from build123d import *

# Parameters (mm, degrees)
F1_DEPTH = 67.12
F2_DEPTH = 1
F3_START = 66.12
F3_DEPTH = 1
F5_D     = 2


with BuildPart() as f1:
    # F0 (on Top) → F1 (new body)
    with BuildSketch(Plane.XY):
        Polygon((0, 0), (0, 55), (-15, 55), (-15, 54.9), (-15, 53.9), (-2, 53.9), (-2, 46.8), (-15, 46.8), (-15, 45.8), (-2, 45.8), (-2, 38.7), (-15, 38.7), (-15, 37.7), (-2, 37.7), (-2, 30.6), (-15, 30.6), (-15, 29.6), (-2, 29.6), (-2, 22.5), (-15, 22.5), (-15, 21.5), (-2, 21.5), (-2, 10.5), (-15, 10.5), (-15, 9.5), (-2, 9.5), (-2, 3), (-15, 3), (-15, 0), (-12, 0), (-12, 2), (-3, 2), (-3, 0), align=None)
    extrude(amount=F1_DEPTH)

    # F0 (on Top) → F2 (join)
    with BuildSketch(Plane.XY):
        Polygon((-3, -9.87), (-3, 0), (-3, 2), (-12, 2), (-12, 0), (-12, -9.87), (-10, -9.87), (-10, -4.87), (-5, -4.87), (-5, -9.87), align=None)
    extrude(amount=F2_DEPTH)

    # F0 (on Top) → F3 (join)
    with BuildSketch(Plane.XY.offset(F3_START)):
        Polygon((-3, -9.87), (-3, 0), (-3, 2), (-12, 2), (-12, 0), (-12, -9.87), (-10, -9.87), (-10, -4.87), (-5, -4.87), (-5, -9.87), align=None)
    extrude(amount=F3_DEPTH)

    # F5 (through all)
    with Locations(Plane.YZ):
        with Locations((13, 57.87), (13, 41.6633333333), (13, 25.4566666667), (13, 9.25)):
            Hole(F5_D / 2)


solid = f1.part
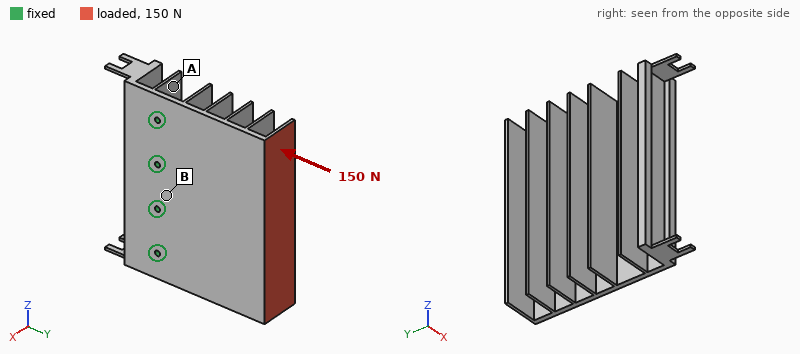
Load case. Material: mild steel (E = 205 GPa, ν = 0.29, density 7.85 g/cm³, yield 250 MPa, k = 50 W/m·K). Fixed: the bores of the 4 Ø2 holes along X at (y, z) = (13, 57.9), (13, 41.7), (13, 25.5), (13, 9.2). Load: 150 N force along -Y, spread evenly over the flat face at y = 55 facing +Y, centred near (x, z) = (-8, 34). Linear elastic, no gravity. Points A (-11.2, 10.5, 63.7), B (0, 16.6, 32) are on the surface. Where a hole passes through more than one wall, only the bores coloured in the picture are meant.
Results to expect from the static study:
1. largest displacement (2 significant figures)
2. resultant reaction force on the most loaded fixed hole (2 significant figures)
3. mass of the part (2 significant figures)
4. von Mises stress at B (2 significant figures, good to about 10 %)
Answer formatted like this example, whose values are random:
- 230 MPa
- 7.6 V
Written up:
- 0.12 mm
- 40 N
- 110 g
- 17 MPa
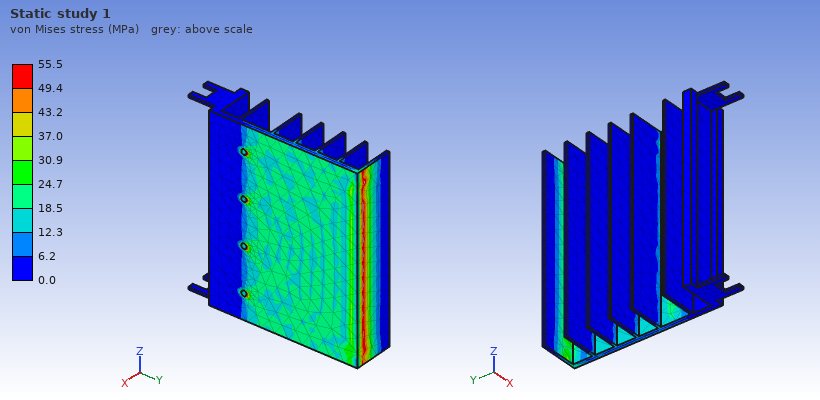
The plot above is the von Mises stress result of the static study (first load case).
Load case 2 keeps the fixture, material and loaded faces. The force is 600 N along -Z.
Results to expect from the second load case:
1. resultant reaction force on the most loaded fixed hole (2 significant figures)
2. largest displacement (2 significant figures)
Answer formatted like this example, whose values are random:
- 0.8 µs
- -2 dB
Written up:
- 500 N
- 0.24 mm
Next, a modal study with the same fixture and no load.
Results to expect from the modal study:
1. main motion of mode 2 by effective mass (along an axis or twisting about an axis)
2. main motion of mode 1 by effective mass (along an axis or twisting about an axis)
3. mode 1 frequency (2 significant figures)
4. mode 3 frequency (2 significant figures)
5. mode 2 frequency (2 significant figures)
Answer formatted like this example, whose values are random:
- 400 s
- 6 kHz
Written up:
- twisting about Y
- along X
- 610 Hz
- 2700 Hz
- 1100 Hz
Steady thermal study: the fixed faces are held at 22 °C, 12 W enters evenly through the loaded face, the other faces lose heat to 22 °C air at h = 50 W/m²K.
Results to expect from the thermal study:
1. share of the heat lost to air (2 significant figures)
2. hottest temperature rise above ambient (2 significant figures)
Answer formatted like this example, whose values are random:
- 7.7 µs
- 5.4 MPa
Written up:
- 80 %
- 47 K
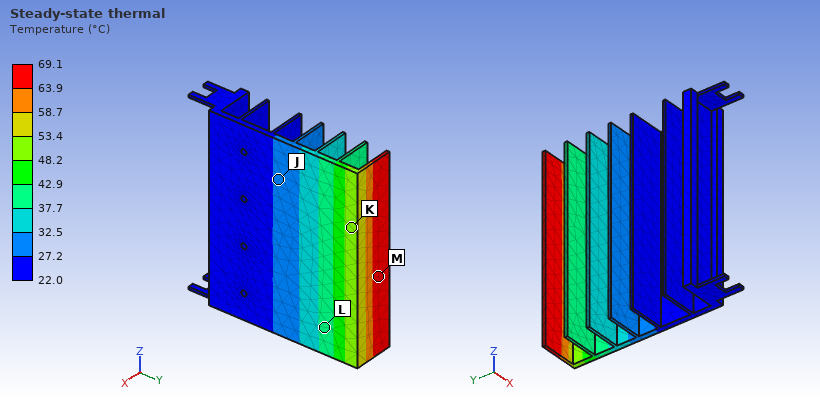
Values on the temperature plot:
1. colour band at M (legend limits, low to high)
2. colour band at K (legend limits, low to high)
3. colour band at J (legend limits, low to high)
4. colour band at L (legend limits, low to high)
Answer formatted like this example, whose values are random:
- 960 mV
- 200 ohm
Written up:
- 63.9 to 69.1 °C
- 48.2 to 53.4 °C
- 27.2 to 32.5 °C
- 37.7 to 42.9 °C
